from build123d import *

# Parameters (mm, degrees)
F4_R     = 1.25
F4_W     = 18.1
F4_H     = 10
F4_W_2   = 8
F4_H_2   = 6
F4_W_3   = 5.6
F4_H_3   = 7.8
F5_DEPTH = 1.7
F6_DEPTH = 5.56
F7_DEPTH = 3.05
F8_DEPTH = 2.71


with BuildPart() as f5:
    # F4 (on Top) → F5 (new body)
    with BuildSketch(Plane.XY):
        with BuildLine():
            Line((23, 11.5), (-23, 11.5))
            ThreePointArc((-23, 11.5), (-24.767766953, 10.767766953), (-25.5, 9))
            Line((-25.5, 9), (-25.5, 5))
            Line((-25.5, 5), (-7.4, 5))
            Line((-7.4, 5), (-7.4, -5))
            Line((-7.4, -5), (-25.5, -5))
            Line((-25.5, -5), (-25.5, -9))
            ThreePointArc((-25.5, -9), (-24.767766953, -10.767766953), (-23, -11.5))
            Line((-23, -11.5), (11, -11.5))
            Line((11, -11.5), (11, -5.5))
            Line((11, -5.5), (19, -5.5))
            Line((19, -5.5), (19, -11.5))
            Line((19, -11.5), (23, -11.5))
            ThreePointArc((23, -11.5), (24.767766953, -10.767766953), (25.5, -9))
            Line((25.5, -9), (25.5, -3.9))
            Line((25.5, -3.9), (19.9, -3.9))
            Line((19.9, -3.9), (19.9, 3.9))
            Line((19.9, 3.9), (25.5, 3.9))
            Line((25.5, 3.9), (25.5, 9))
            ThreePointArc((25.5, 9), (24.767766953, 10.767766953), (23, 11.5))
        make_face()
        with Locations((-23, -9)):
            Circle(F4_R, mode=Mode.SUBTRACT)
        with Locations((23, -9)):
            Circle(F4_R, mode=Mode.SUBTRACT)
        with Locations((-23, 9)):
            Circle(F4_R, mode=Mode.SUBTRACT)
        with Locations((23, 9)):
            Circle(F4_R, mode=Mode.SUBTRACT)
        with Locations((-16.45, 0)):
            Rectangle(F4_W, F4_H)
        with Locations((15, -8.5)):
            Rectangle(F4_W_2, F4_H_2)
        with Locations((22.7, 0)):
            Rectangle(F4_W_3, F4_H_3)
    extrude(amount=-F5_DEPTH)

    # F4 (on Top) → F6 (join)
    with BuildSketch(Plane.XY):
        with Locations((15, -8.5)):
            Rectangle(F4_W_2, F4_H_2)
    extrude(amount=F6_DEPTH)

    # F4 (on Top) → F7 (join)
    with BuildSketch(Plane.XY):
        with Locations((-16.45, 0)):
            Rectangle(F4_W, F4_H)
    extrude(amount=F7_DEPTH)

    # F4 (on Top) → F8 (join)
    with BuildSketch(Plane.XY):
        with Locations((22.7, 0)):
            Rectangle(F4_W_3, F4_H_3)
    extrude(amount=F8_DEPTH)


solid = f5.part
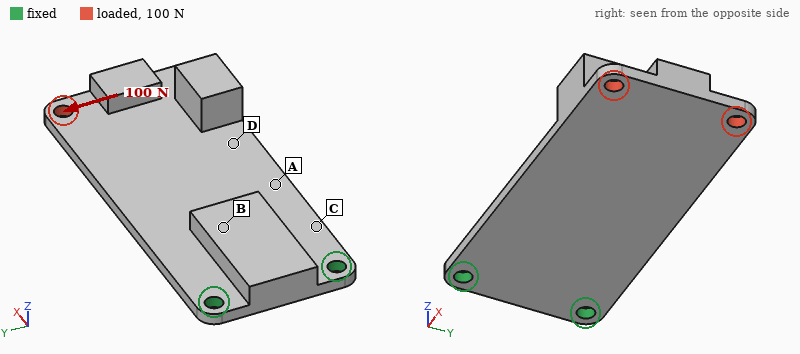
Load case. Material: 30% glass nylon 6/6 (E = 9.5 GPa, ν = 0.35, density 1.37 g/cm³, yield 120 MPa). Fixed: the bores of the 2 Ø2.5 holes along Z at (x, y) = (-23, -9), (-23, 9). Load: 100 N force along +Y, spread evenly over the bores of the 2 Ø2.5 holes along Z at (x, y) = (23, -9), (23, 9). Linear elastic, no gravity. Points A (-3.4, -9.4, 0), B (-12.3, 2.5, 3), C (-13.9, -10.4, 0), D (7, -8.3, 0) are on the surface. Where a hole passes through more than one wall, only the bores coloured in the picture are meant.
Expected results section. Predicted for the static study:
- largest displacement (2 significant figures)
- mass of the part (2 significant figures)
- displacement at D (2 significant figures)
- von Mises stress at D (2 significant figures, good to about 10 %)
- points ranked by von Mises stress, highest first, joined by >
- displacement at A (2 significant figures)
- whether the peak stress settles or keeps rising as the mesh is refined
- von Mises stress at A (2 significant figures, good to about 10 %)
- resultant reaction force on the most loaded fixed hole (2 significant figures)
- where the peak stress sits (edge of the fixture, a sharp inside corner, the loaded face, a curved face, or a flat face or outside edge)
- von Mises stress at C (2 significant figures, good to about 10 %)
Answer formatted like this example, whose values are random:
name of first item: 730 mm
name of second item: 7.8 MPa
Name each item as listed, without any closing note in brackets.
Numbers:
largest displacement: 0.25 mm
mass of the part: 4.0 g
displacement at D: 0.13 mm
von Mises stress at D: 8.5 MPa
points ranked by von Mises stress, highest first, joined by >: C > A > D > B
displacement at A: 0.071 mm
whether the peak stress settles or keeps rising as the mesh is refined: keeps rising
von Mises stress at A: 14 MPa
resultant reaction force on the most loaded fixed hole: 250 N
where the peak stress sits: edge of the fixture
von Mises stress at C: 21 MPa
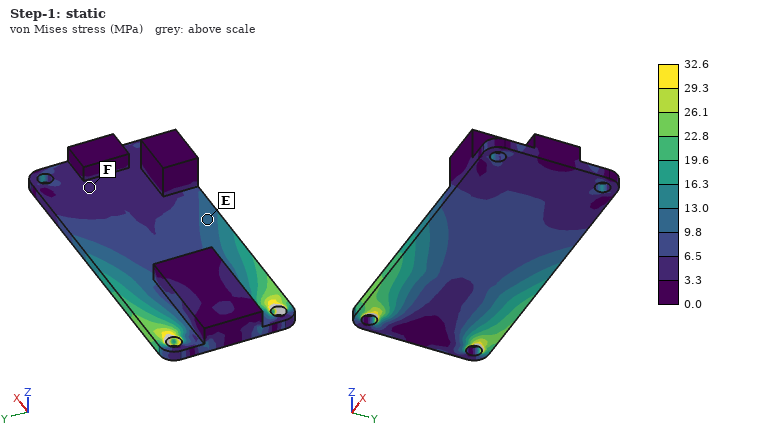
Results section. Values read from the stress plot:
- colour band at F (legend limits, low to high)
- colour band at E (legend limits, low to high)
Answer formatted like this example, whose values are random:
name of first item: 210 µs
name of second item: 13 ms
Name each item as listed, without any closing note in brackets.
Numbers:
colour band at F: 3.3 to 6.5 MPa
colour band at E: 9.8 to 13.0 MPa
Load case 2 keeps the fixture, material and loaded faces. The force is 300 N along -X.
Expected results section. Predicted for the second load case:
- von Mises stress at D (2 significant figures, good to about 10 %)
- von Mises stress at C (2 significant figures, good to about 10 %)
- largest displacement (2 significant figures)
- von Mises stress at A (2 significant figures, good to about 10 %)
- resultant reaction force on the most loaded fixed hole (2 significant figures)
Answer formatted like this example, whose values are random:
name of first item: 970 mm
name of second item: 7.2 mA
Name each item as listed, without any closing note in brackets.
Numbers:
von Mises stress at D: 8.3 MPa
von Mises stress at C: 7.7 MPa
largest displacement: 0.11 mm
von Mises stress at A: 7.3 MPa
resultant reaction force on the most loaded fixed hole: 150 N
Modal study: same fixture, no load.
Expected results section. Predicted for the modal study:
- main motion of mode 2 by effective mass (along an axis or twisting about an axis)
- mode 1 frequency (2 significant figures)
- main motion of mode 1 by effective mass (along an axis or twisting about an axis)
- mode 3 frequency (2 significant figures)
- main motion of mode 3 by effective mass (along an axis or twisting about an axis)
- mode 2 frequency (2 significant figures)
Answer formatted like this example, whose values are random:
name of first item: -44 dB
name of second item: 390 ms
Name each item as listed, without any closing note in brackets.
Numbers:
main motion of mode 2 by effective mass: twisting about X
mode 1 frequency: 360 Hz
main motion of mode 1 by effective mass: along Z
mode 3 frequency: 1800 Hz
main motion of mode 3 by effective mass: along Z
mode 2 frequency: 1500 Hz
